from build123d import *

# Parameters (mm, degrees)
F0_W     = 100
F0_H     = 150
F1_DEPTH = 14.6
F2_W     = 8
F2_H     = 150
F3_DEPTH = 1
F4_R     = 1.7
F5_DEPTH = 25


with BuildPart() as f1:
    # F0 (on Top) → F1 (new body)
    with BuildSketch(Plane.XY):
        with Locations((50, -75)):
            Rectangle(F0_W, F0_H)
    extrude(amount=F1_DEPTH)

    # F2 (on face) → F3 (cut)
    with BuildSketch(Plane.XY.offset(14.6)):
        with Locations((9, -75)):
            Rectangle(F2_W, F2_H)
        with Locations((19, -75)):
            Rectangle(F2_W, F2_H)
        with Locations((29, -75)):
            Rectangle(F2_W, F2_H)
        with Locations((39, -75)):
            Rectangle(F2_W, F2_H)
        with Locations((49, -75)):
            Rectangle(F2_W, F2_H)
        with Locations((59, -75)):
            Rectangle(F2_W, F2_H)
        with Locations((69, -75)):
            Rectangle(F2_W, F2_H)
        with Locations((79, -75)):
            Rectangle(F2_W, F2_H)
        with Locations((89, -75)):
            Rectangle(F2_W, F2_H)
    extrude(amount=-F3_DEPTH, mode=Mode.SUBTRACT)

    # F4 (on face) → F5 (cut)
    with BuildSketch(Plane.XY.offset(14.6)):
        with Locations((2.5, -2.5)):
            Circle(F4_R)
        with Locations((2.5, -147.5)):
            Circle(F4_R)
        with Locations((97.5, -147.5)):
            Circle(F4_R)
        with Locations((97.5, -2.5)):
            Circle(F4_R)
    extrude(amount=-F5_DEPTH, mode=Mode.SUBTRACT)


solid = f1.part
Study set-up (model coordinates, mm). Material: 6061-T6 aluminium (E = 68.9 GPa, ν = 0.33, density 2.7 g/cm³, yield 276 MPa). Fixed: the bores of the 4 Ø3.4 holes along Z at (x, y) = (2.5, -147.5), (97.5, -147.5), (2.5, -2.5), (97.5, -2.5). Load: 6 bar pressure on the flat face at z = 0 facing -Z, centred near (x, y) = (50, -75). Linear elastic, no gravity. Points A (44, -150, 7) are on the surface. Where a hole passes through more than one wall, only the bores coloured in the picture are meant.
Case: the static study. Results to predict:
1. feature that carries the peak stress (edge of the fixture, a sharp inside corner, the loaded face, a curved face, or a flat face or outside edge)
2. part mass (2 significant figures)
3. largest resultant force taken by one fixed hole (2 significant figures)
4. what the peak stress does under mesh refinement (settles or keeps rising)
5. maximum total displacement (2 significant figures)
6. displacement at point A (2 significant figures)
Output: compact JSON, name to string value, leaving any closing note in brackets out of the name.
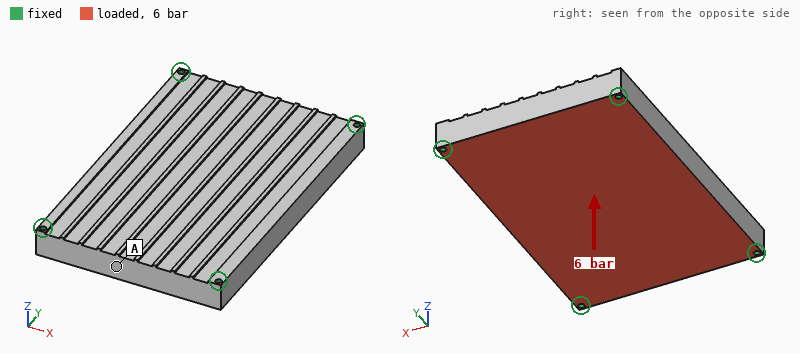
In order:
{"feature that carries the peak stress": "edge of the fixture", "part mass": "560 g", "largest resultant force taken by one fixed hole": "2.3 kN", "what the peak stress does under mesh refinement": "keeps rising", "maximum total displacement": "0.11 mm", "displacement at point A": "0.020 mm"}
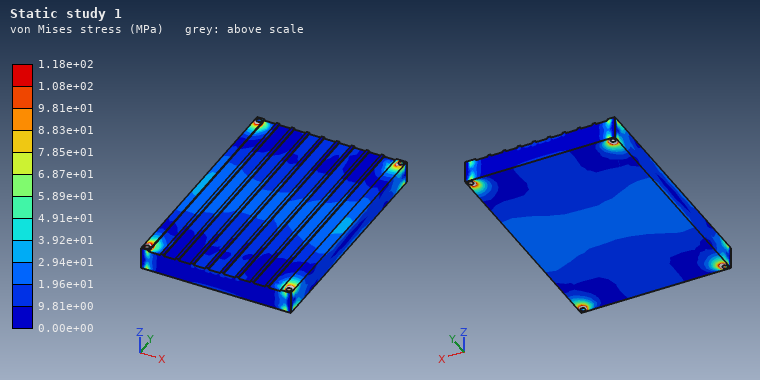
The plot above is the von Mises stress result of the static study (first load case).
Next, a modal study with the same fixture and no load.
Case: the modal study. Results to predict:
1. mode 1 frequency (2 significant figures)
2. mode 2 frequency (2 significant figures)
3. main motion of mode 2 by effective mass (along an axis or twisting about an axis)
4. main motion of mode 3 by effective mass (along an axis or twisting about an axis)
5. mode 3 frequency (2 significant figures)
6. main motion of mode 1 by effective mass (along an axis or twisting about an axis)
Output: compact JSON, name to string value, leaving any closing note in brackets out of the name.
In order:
{"mode 1 frequency": "2200 Hz", "mode 2 frequency": "3800 Hz", "main motion of mode 2 by effective mass": "twisting about Y", "main motion of mode 3 by effective mass": "twisting about X", "mode 3 frequency": "5200 Hz", "main motion of mode 1 by effective mass": "along Z"}
